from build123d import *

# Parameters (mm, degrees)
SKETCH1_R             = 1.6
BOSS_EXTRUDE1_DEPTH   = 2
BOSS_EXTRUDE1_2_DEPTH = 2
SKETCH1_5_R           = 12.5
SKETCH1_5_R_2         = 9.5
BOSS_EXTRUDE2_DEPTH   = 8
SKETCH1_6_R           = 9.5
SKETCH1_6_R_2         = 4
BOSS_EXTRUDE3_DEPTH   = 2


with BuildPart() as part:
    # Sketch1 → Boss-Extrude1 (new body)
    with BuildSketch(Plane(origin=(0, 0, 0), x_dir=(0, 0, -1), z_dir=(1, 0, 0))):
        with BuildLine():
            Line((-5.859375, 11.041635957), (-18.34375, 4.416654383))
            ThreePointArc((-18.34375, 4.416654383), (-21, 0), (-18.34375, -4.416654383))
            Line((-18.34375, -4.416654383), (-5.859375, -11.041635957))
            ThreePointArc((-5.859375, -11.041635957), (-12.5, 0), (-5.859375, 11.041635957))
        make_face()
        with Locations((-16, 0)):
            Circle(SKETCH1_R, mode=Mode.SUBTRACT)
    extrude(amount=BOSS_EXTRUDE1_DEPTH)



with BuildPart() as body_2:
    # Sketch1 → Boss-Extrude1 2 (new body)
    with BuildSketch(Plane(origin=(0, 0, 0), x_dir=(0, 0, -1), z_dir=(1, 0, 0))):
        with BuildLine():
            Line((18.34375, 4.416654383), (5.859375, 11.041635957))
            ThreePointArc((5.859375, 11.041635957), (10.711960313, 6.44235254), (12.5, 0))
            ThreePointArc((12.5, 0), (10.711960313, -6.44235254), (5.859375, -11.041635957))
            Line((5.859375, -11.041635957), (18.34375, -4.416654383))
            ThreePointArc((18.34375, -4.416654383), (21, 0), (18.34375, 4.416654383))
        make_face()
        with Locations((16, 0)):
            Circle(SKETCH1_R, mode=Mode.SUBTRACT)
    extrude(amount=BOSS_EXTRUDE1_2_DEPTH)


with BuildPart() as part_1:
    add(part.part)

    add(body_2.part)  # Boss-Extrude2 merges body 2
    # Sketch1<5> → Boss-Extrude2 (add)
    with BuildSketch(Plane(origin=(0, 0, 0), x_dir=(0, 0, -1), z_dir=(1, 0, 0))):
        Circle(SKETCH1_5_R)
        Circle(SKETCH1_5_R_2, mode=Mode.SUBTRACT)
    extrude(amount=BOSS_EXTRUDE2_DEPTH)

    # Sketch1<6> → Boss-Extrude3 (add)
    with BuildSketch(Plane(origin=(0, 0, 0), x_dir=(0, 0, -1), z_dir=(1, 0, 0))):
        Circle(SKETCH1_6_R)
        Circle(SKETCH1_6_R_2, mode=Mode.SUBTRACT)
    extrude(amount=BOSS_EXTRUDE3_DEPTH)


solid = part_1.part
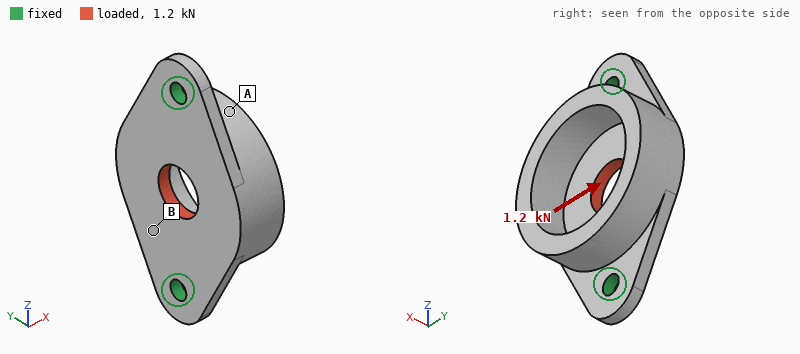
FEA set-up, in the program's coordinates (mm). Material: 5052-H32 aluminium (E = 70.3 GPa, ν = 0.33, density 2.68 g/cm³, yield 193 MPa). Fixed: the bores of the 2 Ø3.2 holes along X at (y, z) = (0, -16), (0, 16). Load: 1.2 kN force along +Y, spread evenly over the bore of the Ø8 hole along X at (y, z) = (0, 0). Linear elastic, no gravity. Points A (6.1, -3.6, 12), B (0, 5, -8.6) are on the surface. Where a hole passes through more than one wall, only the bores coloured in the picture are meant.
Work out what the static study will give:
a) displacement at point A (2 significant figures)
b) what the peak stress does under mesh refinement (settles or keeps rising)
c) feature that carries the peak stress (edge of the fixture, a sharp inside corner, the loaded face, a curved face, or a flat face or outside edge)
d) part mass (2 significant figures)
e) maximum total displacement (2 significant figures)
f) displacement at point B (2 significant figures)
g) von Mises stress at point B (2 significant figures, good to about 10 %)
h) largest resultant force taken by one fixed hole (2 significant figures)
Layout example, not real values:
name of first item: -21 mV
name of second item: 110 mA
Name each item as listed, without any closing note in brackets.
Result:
displacement at point A: 6.0 µm
what the peak stress does under mesh refinement: keeps rising
feature that carries the peak stress: edge of the fixture
part mass: 6.7 g
maximum total displacement: 12 µm
displacement at point B: 7.4 µm
von Mises stress at point B: 20 MPa
largest resultant force taken by one fixed hole: 600 N
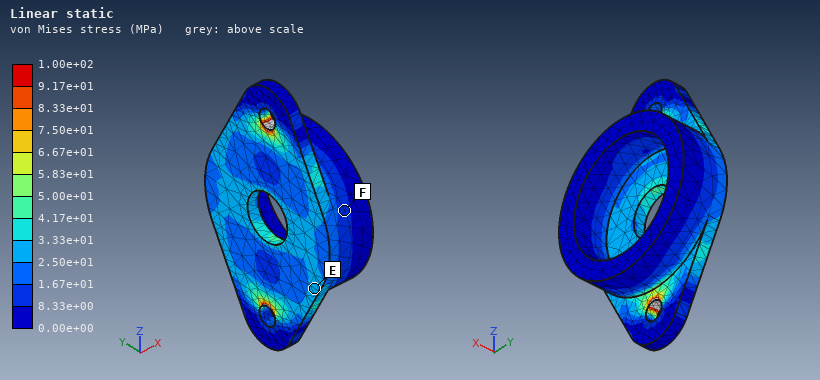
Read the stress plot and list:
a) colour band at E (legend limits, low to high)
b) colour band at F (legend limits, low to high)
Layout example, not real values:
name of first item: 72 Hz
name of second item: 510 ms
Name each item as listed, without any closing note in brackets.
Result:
colour band at E: 2.50e+01 to 3.33e+01 MPa
colour band at F: 8.33e+00 to 1.67e+01 MPa
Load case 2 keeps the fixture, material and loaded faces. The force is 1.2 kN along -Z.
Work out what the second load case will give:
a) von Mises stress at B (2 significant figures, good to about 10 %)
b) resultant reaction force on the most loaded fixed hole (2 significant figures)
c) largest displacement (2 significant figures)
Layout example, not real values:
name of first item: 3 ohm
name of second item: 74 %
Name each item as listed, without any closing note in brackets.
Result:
von Mises stress at B: 18 MPa
resultant reaction force on the most loaded fixed hole: 600 N
largest displacement: 5.6 µm
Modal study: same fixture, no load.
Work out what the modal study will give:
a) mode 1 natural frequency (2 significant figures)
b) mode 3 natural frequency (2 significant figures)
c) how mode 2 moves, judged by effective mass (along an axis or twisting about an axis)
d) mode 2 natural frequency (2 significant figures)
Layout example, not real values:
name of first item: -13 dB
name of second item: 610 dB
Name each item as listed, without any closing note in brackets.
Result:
mode 1 natural frequency: 6300 Hz
mode 3 natural frequency: 24 kHz
how mode 2 moves, judged by effective mass: along X
mode 2 natural frequency: 11 kHz
